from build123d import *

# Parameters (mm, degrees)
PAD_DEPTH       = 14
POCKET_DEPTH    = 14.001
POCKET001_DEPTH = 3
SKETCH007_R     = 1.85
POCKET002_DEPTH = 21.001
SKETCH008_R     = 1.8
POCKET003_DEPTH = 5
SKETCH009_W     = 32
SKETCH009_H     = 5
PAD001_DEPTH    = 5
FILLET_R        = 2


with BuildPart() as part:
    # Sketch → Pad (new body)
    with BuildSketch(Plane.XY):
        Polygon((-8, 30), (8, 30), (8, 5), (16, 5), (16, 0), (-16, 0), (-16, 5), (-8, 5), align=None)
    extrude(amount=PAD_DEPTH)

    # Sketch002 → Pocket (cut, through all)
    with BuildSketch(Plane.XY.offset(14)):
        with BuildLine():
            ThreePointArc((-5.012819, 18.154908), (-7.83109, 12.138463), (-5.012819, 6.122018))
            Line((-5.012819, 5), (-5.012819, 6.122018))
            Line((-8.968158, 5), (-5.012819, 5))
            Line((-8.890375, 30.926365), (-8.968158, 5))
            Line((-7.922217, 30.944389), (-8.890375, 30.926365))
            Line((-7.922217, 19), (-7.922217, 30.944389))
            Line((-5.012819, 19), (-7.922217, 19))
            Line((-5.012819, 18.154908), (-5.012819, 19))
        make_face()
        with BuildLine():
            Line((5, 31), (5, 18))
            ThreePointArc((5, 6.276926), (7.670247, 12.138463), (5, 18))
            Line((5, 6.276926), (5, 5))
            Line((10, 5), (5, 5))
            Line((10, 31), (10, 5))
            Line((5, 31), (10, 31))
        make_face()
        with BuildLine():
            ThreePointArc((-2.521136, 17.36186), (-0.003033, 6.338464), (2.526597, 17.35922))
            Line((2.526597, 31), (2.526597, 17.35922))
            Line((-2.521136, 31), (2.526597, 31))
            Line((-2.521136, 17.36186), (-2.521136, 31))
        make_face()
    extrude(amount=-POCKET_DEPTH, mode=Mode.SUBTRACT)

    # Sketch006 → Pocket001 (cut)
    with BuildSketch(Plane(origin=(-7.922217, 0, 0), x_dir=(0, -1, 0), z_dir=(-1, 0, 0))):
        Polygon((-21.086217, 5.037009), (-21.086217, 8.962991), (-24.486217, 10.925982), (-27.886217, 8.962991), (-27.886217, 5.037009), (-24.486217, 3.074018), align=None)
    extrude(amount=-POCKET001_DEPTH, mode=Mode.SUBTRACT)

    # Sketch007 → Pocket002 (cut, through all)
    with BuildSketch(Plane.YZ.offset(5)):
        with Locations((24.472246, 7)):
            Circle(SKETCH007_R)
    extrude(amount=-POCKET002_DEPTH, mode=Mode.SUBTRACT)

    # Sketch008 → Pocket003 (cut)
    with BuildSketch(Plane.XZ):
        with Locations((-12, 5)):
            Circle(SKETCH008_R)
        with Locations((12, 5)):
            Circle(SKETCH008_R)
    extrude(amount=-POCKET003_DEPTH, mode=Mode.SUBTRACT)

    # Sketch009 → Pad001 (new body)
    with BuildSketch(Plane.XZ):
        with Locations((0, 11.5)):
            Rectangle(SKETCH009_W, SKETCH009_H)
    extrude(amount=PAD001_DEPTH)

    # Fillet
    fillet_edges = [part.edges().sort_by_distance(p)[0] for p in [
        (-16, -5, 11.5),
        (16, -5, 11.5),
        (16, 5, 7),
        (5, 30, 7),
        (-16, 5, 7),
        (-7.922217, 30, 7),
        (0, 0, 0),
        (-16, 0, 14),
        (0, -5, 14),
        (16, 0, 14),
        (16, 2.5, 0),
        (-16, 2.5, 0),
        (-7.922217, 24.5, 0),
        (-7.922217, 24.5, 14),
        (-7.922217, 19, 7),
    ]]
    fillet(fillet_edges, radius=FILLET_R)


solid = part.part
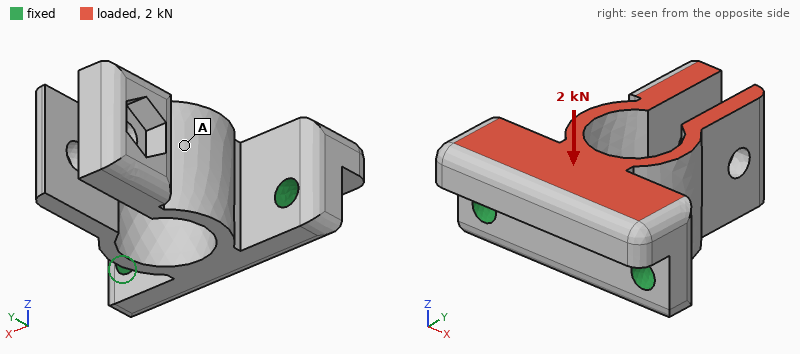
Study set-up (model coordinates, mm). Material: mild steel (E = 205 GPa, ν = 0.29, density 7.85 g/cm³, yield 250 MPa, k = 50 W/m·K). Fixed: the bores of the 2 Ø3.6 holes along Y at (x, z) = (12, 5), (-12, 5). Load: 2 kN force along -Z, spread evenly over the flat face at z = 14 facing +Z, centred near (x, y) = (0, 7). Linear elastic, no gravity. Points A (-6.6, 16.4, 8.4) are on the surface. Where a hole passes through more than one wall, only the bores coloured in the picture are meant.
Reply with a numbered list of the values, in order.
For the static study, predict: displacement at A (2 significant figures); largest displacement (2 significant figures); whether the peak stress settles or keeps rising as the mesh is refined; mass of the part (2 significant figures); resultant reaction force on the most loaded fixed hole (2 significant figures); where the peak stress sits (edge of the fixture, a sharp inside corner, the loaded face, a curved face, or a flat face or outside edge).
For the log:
1. 24 µm
2. 66 µm
3. keeps rising
4. 38 g
5. 1.1 kN
6. a sharp inside corner
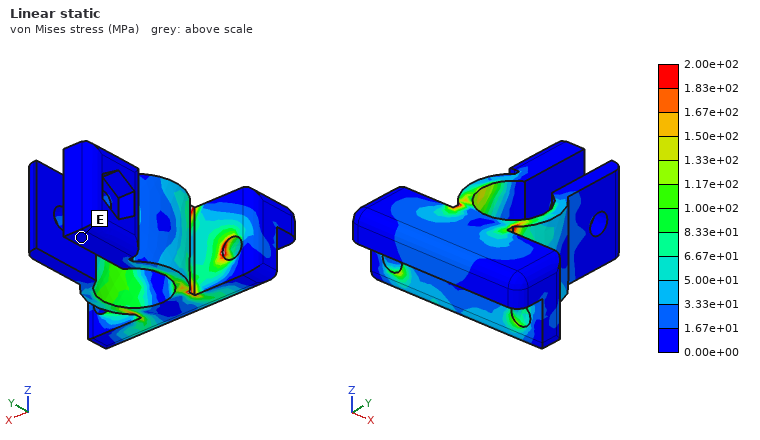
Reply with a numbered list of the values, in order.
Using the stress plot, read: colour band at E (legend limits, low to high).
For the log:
1. 0.00e+00 to 1.67e+01 MPa
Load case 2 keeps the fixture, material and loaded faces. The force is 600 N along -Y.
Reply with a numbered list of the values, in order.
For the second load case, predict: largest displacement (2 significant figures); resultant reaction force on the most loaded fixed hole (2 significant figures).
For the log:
1. 22 µm
2. 310 N
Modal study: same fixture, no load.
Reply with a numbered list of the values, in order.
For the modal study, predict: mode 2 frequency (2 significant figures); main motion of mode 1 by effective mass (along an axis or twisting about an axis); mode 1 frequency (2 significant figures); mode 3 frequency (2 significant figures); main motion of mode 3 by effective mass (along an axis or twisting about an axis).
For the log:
1. 2400 Hz
2. along X
3. 2000 Hz
4. 5000 Hz
5. along Z
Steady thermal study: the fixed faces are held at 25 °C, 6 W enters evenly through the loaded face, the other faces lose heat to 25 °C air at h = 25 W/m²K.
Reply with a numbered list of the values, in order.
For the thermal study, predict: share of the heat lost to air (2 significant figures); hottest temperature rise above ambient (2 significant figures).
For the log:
1. 9.9 %
2. 15 K
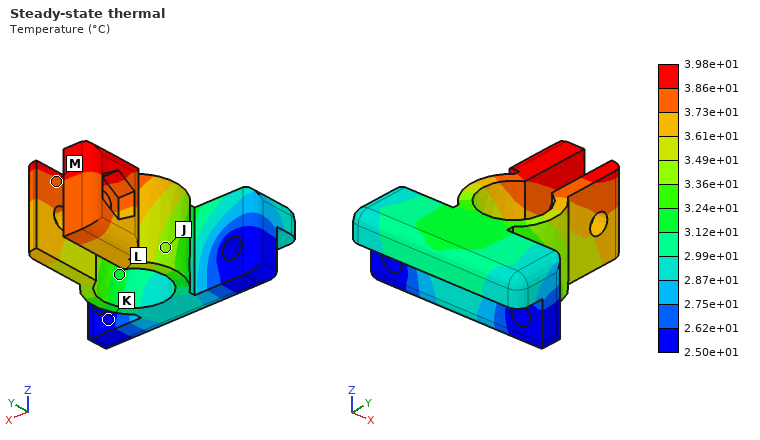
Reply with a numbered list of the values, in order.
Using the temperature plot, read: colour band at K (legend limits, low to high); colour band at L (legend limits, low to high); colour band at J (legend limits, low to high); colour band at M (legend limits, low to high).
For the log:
1. 2.50e+01 to 2.62e+01 °C
2. 3.12e+01 to 3.24e+01 °C
3. 3.36e+01 to 3.49e+01 °C
4. 3.73e+01 to 3.86e+01 °C
